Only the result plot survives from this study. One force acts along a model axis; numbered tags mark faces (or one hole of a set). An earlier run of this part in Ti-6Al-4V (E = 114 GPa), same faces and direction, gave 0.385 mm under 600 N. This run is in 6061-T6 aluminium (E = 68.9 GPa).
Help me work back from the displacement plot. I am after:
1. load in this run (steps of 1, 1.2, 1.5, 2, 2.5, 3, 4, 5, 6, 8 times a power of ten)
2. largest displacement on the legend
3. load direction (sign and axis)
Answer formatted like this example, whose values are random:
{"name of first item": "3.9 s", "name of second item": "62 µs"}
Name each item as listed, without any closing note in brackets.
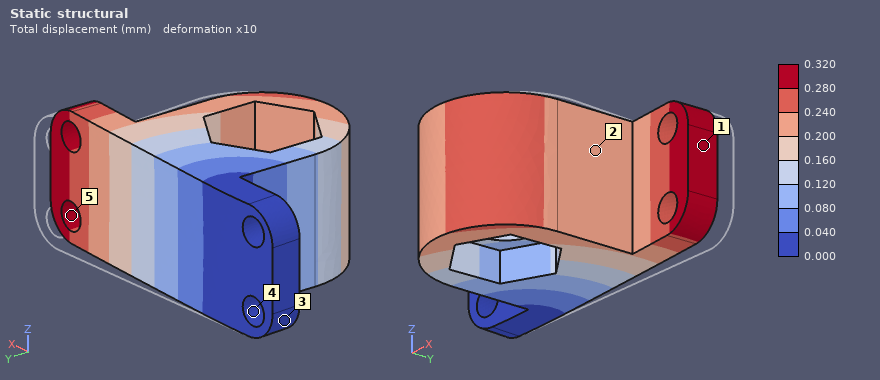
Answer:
{"load in this run": "300 N", "largest displacement on the legend": "0.320 mm", "load direction": "-Y"}
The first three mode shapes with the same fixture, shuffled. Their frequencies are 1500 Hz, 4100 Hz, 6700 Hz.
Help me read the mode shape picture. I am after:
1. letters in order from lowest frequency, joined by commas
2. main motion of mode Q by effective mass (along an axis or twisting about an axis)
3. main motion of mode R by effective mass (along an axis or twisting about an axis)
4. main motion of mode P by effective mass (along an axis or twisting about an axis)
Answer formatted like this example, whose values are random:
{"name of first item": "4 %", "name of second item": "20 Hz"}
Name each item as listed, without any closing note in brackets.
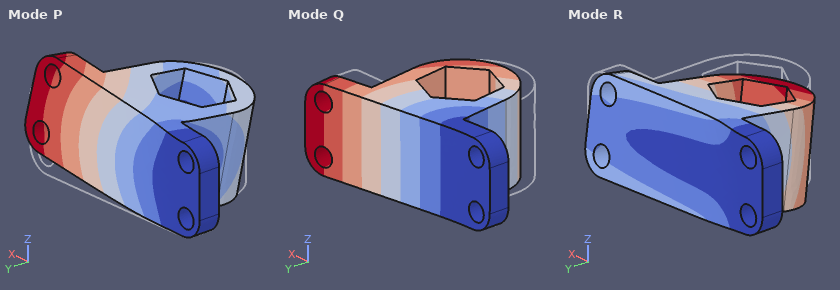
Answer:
{"letters in order from lowest frequency, joined by commas": "Q, R, P", "main motion of mode Q by effective mass": "along Y", "main motion of mode R by effective mass": "along Z", "main motion of mode P by effective mass": "along Z"}
